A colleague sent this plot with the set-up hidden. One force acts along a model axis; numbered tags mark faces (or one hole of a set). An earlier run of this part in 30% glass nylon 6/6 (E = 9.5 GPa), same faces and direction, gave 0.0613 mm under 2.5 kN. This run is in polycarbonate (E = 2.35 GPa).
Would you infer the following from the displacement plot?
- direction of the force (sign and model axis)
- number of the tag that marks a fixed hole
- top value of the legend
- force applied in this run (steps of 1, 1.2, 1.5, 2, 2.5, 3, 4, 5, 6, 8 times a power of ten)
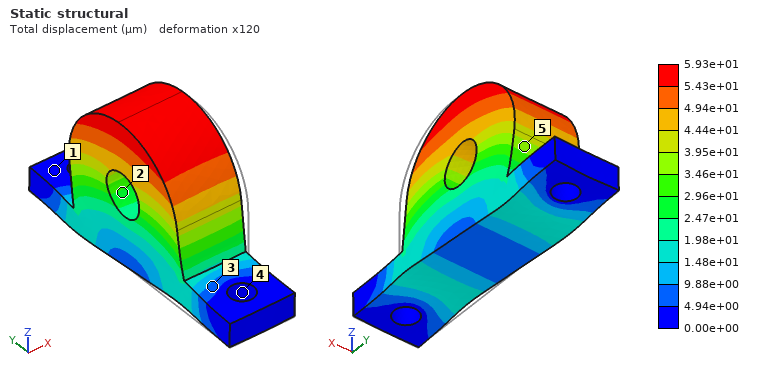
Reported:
+Y
4
5.93e+01 µm
600 N
